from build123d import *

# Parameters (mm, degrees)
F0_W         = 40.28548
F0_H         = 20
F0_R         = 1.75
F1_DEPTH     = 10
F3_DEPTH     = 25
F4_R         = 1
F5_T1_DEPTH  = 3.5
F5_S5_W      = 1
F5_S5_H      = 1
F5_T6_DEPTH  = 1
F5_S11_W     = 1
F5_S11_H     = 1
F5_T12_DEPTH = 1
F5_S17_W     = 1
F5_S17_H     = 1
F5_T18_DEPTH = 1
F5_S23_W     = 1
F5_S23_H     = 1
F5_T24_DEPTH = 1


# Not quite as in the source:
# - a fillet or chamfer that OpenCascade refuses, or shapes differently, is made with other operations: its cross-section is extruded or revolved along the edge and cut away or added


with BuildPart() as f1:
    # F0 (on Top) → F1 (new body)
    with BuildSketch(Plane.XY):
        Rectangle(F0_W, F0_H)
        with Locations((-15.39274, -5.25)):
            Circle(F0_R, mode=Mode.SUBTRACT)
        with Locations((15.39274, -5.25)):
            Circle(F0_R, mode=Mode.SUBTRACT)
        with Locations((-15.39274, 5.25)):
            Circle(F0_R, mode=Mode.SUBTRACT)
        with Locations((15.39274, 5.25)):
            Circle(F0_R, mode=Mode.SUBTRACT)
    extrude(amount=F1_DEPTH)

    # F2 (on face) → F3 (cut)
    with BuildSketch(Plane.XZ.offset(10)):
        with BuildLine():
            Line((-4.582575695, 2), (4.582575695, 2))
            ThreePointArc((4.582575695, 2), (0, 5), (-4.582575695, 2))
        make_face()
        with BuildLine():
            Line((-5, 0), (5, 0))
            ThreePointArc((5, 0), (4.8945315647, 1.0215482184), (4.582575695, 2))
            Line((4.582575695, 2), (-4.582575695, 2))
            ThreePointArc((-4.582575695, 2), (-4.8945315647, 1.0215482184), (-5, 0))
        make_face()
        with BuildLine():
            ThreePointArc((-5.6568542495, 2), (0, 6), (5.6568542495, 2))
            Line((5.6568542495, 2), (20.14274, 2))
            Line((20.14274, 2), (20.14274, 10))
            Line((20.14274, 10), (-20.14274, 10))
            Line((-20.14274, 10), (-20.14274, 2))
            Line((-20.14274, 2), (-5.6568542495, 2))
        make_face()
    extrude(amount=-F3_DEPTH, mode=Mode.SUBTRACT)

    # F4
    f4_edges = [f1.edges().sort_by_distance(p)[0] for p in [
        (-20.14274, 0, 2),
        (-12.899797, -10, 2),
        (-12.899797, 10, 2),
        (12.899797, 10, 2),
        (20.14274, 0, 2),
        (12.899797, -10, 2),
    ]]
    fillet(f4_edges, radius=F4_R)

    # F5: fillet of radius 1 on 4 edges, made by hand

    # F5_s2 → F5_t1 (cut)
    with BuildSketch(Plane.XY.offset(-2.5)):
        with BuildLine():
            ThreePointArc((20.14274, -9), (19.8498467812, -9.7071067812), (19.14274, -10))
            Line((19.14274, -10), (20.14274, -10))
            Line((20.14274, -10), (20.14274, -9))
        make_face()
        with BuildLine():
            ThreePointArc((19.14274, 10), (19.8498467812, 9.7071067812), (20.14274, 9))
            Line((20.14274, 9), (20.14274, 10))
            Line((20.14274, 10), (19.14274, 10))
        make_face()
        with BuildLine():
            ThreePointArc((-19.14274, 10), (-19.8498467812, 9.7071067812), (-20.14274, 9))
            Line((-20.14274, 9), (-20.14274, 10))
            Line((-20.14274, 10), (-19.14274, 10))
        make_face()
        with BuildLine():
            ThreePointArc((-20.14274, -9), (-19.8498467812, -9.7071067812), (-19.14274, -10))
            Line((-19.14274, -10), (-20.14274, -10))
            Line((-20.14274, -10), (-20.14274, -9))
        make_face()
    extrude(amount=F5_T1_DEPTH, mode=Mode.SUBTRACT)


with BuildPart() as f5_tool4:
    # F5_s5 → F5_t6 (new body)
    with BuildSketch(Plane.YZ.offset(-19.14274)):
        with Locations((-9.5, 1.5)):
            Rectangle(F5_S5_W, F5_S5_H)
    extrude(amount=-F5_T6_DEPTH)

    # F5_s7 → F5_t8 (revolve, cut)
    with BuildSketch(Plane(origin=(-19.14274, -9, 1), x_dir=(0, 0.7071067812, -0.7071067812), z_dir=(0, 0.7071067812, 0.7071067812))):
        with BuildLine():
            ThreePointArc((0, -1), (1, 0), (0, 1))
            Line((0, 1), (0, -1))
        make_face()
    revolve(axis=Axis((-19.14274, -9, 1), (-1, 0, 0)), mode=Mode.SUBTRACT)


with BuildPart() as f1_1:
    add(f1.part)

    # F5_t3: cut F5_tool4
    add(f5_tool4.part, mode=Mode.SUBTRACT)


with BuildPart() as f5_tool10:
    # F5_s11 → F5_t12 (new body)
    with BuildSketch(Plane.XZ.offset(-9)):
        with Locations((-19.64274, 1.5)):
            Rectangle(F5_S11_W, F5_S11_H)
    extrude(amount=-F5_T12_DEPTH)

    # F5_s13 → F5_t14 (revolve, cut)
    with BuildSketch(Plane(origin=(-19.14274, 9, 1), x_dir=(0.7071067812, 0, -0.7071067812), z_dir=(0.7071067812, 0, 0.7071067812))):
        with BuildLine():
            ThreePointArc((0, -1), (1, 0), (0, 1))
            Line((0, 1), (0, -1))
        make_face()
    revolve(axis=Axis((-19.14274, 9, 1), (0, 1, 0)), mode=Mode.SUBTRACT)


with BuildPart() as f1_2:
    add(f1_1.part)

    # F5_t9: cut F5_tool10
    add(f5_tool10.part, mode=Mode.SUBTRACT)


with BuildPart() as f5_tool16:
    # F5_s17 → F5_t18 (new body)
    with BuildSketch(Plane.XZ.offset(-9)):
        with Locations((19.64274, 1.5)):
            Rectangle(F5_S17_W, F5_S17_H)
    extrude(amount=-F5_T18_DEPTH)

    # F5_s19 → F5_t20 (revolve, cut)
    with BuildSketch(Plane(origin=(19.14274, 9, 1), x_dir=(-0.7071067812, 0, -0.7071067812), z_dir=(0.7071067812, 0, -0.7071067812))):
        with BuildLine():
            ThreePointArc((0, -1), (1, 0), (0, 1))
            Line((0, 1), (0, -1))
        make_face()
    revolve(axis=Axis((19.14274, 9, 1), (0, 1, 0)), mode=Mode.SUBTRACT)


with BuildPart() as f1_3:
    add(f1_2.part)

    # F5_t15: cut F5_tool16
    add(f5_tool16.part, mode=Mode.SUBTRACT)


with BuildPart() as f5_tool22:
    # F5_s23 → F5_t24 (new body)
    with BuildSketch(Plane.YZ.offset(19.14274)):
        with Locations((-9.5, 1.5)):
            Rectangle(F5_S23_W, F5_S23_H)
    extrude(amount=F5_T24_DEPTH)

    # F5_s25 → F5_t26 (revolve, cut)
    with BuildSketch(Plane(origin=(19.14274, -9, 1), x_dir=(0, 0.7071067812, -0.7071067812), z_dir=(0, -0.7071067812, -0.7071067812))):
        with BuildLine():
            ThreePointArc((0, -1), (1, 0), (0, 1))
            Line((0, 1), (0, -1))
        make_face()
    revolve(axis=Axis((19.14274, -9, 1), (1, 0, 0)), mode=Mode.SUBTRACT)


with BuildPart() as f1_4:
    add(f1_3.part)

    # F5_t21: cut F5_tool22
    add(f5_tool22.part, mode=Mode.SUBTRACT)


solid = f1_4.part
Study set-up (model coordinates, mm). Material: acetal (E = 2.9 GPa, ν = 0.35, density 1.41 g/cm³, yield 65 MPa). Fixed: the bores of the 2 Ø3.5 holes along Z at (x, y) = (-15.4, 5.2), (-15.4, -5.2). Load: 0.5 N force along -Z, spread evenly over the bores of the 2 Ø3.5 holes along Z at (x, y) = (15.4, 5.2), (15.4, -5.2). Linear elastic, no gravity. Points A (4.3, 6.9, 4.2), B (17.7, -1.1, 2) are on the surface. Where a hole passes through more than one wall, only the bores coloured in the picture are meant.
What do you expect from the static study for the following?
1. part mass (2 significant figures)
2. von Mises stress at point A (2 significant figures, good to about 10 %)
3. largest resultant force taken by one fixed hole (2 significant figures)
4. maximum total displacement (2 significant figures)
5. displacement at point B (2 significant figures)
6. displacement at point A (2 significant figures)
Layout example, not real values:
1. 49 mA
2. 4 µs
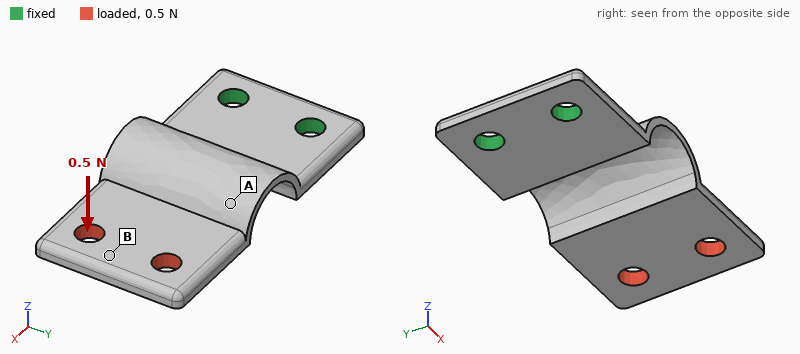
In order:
1. 2.0 g
2. 1.4 MPa
3. 0.28 N
4. 0.52 mm
5. 0.46 mm
6. 0.14 mm
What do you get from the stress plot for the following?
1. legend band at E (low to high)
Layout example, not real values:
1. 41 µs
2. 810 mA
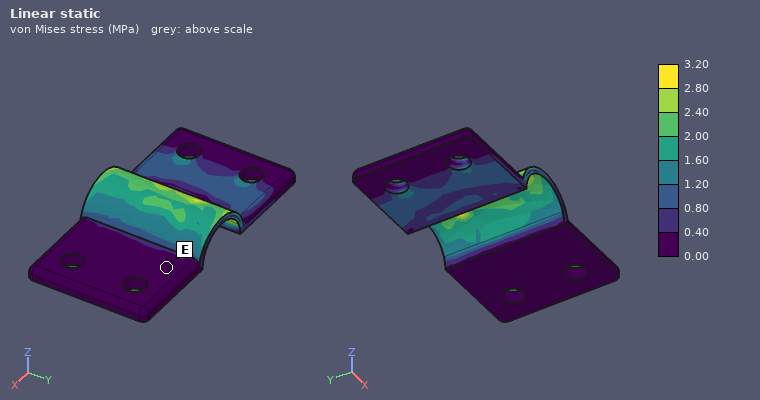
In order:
1. 0.00 to 0.40 MPa
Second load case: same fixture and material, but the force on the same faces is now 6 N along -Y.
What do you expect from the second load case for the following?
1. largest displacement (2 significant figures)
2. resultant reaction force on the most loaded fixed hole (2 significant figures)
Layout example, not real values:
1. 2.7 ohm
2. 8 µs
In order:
1. 0.53 mm
2. 15 N
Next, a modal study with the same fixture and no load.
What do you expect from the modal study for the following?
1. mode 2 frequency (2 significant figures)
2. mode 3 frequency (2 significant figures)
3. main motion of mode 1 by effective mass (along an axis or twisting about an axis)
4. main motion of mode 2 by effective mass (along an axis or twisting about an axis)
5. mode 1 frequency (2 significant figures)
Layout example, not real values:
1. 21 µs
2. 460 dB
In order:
1. 660 Hz
2. 1200 Hz
3. along Z
4. along Y
5. 220 Hz
